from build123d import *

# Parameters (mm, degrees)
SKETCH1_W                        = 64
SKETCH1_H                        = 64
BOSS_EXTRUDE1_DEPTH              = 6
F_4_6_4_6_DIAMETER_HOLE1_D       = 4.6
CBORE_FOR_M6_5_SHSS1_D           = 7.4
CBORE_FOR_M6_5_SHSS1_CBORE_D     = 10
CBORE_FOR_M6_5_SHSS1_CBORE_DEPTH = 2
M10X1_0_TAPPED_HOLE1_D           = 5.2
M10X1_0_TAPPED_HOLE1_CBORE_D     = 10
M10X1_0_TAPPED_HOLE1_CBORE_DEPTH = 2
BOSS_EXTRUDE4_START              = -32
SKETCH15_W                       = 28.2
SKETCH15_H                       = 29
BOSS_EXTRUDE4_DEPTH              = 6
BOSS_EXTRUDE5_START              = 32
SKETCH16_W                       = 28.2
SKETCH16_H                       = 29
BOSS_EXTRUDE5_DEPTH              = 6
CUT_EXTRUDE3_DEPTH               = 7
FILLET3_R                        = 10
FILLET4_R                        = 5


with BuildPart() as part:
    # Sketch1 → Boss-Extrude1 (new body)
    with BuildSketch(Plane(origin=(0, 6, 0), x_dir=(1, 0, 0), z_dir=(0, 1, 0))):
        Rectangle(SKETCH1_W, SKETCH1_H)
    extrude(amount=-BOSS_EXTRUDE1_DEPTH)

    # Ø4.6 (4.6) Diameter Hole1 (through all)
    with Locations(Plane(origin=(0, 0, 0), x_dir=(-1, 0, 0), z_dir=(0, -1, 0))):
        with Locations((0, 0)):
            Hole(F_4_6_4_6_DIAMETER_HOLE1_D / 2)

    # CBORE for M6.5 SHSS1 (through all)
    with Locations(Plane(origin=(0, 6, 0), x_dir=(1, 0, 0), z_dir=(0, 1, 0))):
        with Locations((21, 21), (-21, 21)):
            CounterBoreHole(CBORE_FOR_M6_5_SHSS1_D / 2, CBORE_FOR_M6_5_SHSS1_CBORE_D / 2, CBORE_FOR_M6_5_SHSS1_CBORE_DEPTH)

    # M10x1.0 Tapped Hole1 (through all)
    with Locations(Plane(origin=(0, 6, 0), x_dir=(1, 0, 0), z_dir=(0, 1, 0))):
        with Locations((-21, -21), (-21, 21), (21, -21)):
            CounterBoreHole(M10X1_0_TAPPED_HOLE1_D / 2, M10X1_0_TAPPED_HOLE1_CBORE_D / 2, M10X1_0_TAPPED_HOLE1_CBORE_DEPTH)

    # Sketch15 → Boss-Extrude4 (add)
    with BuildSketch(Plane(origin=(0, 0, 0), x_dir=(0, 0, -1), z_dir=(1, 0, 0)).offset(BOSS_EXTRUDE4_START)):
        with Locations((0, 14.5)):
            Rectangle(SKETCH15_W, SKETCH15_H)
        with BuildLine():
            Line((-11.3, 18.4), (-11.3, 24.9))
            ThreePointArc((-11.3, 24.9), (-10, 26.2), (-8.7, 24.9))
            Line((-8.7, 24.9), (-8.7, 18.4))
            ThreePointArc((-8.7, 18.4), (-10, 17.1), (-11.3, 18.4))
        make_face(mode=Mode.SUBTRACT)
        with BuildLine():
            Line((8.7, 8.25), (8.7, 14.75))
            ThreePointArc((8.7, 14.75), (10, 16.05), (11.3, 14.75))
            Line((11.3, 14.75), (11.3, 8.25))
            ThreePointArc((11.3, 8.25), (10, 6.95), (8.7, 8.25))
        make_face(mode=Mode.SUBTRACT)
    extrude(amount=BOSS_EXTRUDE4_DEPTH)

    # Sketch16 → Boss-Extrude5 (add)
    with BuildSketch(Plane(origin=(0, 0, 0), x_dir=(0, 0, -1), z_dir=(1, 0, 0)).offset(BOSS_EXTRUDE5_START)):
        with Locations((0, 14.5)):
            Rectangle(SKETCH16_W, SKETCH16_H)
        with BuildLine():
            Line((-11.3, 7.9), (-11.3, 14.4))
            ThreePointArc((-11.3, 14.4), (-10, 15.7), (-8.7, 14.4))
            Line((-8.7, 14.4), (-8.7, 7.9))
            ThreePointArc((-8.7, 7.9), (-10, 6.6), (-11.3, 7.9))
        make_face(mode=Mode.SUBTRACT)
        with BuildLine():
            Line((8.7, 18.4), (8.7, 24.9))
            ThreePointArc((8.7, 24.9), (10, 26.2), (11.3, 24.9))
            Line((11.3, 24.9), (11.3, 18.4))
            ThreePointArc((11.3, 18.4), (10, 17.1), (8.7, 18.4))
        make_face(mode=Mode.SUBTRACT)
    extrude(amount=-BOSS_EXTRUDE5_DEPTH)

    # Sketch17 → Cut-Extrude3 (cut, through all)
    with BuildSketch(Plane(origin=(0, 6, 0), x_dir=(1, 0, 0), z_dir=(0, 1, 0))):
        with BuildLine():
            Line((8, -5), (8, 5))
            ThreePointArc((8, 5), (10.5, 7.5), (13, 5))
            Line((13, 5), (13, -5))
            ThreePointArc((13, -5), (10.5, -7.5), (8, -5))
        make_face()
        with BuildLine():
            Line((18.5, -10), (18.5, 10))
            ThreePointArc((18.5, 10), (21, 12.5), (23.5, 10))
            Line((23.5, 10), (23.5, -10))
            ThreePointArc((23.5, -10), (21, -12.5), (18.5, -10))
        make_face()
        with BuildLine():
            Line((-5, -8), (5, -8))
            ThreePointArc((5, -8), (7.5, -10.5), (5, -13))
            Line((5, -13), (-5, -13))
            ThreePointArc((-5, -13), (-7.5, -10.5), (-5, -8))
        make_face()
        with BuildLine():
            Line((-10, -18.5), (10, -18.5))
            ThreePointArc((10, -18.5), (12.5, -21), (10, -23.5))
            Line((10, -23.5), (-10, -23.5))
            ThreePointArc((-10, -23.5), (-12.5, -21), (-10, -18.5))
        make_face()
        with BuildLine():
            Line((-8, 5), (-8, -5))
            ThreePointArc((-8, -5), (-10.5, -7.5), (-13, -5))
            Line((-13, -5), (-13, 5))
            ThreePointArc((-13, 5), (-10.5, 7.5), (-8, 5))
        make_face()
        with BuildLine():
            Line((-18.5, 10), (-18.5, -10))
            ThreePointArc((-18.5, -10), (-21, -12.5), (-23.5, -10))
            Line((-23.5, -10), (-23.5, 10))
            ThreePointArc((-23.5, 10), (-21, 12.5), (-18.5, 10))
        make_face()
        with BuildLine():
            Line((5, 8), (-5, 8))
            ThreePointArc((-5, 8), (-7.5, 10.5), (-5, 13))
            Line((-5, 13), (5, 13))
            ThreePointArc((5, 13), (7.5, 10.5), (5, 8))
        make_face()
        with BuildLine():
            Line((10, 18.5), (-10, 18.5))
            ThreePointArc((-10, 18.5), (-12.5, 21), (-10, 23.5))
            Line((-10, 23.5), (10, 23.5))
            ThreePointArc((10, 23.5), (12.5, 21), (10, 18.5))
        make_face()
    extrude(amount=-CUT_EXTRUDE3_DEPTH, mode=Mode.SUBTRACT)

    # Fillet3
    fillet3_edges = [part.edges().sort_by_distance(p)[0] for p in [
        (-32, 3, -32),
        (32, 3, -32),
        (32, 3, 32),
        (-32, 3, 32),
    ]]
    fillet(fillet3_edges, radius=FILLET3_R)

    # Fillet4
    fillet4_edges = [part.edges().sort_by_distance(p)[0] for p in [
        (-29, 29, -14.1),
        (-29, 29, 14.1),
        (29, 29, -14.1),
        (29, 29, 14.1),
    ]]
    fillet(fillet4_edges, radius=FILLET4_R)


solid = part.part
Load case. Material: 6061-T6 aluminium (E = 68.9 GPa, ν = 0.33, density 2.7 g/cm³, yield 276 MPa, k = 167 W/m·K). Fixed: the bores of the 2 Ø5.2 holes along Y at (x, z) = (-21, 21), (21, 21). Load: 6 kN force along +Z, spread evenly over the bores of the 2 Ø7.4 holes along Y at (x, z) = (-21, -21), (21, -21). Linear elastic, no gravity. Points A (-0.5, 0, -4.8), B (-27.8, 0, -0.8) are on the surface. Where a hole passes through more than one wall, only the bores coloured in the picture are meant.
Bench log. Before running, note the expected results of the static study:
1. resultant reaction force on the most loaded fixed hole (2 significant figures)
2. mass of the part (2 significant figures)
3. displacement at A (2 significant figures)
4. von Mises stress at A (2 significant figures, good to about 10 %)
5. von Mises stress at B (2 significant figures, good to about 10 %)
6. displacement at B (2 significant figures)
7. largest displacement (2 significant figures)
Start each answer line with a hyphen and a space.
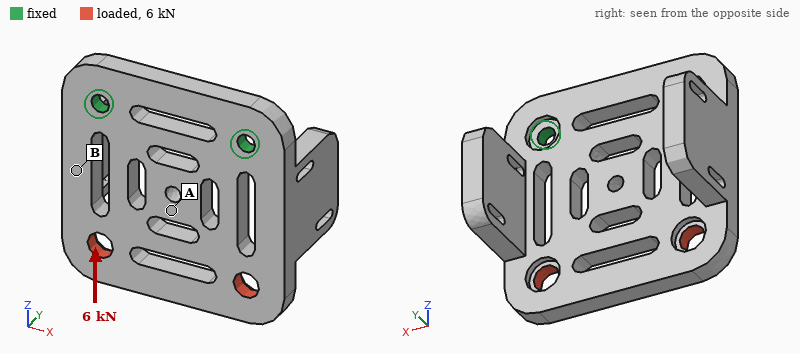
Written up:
- 3.0 kN
- 69 g
- 0.029 mm
- 10 MPa
- 34 MPa
- 0.028 mm
- 0.12 mm
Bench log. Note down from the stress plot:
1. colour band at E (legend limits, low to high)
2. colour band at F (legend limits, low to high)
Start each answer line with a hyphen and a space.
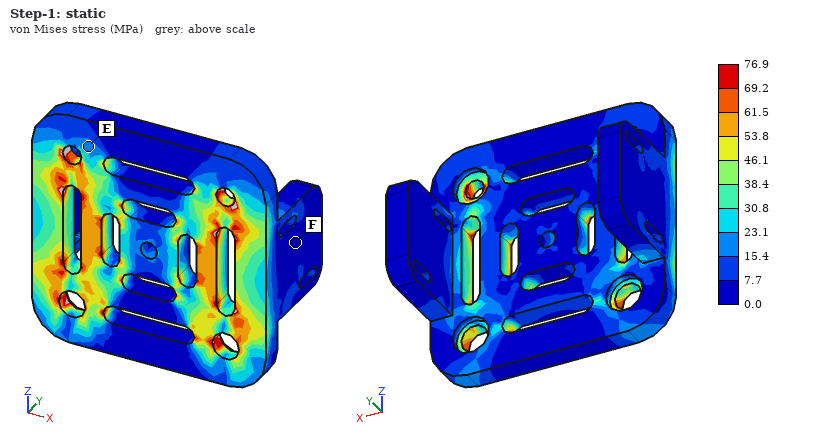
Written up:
- 15.4 to 23.1 MPa
- 0.0 to 7.7 MPa
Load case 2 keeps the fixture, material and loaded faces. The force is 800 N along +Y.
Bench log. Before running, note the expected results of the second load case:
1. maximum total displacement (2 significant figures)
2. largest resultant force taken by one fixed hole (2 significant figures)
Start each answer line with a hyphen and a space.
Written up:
- 0.57 mm
- 410 N
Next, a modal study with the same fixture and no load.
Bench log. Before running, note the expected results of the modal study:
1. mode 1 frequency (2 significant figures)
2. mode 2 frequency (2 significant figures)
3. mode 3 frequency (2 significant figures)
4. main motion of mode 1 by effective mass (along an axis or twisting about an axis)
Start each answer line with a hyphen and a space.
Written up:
- 1300 Hz
- 2100 Hz
- 3300 Hz
- along Y
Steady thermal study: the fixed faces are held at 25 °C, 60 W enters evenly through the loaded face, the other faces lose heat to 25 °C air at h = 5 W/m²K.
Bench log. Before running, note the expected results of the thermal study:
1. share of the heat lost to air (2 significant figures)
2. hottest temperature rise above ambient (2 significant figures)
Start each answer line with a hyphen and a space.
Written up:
- 3.5 %
- 67 K
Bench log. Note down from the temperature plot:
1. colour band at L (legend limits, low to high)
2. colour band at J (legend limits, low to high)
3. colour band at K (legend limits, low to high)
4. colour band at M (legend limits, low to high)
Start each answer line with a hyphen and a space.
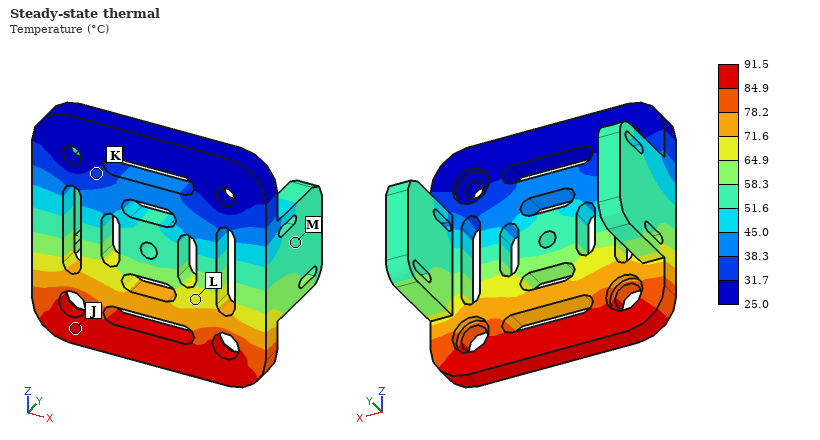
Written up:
- 64.9 to 71.6 °C
- 84.9 to 91.5 °C
- 31.7 to 38.3 °C
- 51.6 to 58.3 °C
